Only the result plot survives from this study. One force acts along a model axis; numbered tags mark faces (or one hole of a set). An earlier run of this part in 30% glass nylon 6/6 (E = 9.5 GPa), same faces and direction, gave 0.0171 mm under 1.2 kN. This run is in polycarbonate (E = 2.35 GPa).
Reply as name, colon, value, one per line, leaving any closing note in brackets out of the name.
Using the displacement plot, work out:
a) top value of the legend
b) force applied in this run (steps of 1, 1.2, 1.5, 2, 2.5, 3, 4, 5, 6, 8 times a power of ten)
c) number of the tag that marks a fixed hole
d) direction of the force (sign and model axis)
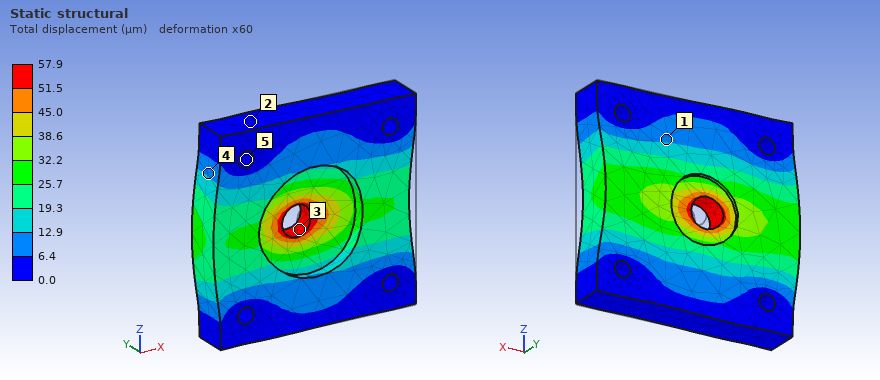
top value of the legend: 57.9 µm
force applied in this run: 1 kN
number of the tag that marks a fixed hole: 5
direction of the force: -X
